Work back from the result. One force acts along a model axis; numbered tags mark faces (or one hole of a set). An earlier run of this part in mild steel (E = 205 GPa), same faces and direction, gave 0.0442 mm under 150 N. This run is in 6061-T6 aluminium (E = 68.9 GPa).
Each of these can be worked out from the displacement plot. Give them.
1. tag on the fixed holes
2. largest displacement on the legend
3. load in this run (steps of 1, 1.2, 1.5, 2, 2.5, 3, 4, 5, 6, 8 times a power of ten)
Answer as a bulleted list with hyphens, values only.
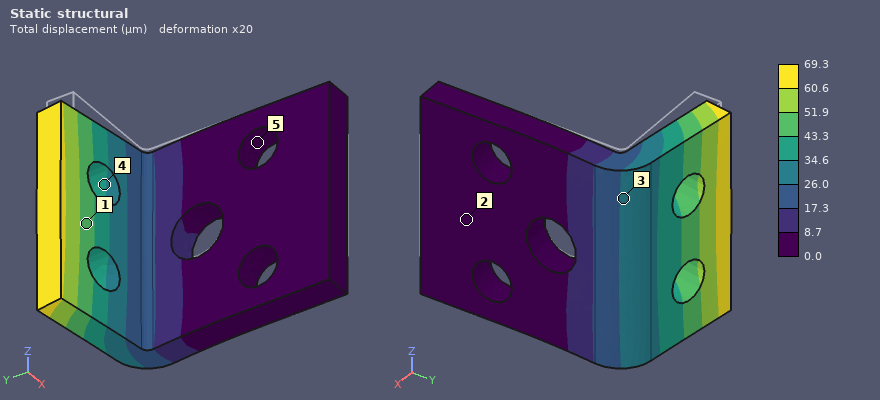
- 5
- 69.3 µm
- 80 N
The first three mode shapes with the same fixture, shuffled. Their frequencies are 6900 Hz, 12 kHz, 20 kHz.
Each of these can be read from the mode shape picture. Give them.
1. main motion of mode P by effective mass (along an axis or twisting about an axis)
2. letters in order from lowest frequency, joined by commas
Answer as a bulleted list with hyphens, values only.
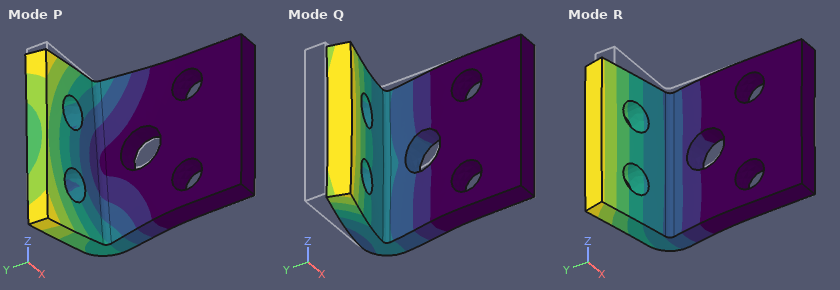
- along Z
- R, P, Q
